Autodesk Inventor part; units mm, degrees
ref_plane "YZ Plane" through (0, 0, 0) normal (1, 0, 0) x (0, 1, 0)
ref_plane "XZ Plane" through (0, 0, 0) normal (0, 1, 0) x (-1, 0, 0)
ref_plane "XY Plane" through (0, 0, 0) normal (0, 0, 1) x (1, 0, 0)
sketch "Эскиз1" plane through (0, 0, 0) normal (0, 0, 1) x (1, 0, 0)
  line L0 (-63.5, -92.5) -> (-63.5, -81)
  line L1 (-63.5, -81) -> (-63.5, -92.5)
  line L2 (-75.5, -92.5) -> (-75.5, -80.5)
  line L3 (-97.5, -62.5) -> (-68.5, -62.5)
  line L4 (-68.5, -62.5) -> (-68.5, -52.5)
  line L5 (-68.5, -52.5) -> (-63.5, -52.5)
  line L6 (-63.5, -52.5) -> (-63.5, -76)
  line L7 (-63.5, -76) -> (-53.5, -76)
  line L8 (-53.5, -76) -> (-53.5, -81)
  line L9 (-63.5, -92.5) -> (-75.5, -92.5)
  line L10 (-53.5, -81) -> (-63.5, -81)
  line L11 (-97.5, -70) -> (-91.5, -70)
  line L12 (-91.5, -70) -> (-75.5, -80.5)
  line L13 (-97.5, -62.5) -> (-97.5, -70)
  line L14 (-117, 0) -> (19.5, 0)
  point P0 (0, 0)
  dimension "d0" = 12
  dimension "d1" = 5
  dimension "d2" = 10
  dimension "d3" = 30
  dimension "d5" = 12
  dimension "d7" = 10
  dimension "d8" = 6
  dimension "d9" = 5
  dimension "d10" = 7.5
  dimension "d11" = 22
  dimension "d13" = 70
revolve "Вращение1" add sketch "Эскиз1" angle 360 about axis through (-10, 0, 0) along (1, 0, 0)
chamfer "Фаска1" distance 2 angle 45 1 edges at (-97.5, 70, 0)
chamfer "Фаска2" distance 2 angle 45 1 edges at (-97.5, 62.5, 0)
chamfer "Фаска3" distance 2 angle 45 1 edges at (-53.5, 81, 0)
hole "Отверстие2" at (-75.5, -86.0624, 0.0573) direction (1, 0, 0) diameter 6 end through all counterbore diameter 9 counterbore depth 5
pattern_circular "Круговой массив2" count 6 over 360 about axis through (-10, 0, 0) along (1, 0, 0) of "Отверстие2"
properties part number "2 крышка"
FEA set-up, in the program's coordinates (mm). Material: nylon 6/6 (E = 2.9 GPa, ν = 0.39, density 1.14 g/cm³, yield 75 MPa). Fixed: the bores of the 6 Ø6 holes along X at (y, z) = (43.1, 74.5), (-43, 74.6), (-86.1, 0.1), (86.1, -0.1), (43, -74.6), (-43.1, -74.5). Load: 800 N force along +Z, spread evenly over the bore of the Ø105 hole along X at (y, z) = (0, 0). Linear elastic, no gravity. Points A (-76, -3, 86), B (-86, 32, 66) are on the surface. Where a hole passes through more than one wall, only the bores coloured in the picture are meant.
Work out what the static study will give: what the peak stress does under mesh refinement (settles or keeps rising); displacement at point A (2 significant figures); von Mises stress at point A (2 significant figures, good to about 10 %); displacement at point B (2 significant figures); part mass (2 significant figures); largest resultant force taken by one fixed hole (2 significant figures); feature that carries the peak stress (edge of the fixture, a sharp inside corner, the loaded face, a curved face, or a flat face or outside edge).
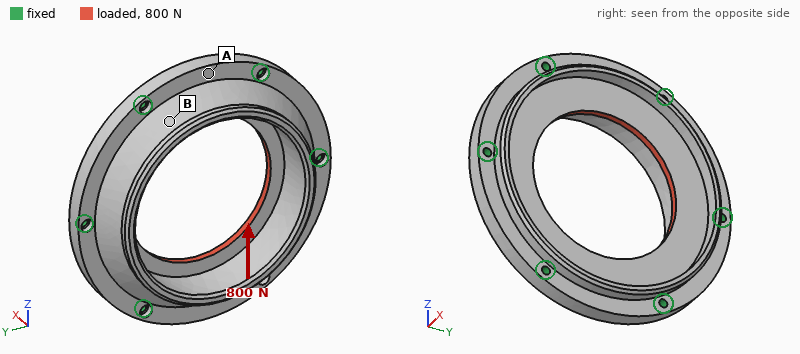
keeps rising
7.8 µm
0.30 MPa
3.1 µm
360 g
150 N
edge of the fixture
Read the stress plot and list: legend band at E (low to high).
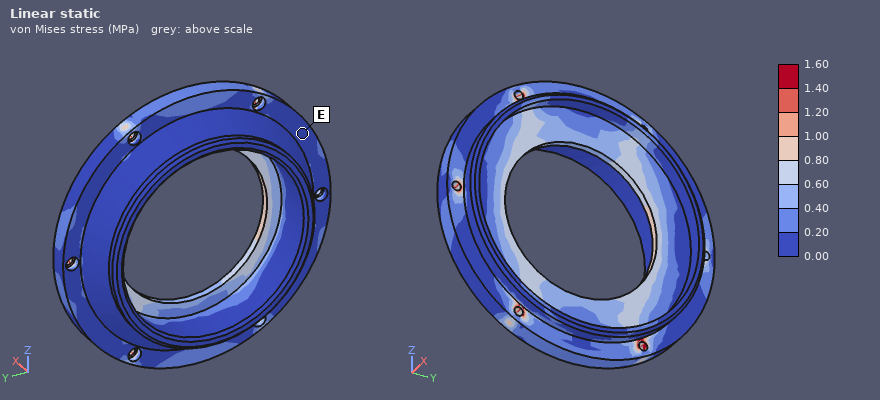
0.00 to 0.20 MPa
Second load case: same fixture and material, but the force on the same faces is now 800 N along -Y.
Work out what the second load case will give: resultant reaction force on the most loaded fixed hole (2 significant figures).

160 N
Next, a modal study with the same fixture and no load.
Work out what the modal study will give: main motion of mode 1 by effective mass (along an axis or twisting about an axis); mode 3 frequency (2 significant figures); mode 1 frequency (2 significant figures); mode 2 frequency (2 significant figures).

along X
2200 Hz
2000 Hz
2200 Hz
